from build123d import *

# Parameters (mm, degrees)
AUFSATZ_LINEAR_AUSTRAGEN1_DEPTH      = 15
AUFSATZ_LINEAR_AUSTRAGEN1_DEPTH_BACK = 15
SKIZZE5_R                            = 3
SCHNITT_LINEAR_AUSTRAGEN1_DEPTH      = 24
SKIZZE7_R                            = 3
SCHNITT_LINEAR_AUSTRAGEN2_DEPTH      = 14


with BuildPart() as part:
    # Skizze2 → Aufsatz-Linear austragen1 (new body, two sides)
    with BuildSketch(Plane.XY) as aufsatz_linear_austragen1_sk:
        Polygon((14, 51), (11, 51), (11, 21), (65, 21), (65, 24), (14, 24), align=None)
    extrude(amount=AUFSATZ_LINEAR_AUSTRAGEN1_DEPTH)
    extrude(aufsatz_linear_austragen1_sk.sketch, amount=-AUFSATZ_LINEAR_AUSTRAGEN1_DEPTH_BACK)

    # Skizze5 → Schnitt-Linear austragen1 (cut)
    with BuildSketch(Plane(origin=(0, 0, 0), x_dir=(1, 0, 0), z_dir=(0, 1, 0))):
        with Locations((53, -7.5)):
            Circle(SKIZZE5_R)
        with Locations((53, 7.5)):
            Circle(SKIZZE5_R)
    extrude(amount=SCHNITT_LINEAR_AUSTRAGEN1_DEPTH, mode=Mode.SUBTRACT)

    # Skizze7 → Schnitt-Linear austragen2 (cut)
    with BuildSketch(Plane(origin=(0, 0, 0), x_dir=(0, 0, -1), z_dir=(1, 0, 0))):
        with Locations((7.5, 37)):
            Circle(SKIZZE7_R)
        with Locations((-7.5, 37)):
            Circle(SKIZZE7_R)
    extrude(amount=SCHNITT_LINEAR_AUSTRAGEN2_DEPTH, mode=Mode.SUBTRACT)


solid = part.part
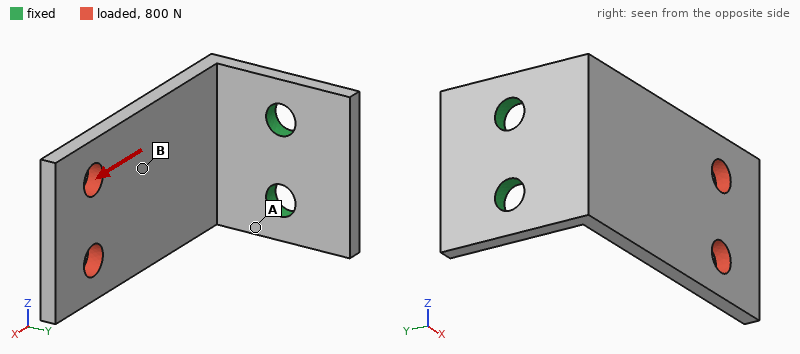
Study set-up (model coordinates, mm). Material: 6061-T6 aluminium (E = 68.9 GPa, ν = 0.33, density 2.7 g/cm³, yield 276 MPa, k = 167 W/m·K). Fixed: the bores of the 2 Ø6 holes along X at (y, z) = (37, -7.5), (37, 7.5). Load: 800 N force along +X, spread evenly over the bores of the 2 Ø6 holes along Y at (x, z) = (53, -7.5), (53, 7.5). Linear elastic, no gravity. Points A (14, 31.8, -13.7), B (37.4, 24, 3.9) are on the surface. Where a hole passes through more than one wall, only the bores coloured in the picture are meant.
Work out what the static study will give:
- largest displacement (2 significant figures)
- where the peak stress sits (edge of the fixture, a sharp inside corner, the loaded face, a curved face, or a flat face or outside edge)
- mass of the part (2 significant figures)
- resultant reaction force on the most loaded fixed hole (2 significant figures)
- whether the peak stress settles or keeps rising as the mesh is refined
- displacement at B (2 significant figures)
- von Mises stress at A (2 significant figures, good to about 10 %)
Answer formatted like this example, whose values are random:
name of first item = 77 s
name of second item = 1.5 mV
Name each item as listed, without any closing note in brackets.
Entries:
largest displacement = 0.69 mm
where the peak stress sits = edge of the fixture
mass of the part = 19 g
resultant reaction force on the most loaded fixed hole = 400 N
whether the peak stress settles or keeps rising as the mesh is refined = keeps rising
displacement at B = 0.33 mm
von Mises stress at A = 130 MPa
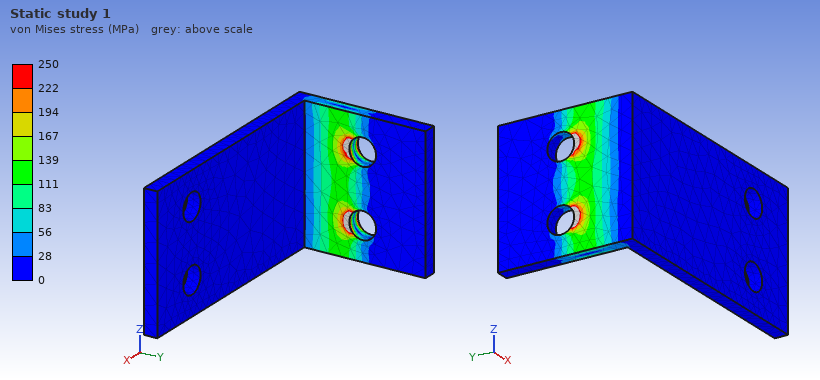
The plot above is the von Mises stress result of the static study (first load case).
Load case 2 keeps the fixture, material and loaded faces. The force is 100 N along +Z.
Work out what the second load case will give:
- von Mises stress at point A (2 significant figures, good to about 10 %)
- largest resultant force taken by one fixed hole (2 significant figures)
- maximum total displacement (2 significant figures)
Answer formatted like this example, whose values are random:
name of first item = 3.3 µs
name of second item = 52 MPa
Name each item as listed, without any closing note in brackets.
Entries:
von Mises stress at point A = 37 MPa
largest resultant force taken by one fixed hole = 220 N
maximum total displacement = 0.16 mm
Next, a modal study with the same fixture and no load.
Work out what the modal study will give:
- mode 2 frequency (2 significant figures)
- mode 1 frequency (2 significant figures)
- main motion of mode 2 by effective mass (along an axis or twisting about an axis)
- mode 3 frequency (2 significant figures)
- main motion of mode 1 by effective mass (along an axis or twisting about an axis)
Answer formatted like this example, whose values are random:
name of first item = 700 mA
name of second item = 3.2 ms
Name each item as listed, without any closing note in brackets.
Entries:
mode 2 frequency = 1700 Hz
mode 1 frequency = 690 Hz
main motion of mode 2 by effective mass = along Z
mode 3 frequency = 3300 Hz
main motion of mode 1 by effective mass = along Y
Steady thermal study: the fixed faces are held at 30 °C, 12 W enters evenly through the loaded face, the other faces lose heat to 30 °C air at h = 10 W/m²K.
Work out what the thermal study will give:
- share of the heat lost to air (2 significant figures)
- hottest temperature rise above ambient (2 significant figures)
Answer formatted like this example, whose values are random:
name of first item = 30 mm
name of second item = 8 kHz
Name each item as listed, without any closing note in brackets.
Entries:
share of the heat lost to air = 8.2 %
hottest temperature rise above ambient = 42 K
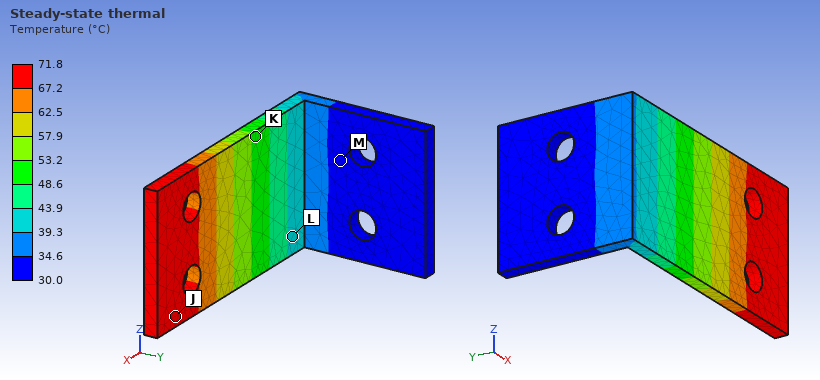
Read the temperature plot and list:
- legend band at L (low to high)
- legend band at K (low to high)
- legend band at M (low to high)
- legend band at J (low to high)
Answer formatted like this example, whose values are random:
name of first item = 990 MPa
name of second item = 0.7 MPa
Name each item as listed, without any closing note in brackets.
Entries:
legend band at L = 39.3 to 43.9 °C
legend band at K = 48.6 to 53.2 °C
legend band at M = 30.0 to 34.6 °C
legend band at J = 67.2 to 71.8 °C
